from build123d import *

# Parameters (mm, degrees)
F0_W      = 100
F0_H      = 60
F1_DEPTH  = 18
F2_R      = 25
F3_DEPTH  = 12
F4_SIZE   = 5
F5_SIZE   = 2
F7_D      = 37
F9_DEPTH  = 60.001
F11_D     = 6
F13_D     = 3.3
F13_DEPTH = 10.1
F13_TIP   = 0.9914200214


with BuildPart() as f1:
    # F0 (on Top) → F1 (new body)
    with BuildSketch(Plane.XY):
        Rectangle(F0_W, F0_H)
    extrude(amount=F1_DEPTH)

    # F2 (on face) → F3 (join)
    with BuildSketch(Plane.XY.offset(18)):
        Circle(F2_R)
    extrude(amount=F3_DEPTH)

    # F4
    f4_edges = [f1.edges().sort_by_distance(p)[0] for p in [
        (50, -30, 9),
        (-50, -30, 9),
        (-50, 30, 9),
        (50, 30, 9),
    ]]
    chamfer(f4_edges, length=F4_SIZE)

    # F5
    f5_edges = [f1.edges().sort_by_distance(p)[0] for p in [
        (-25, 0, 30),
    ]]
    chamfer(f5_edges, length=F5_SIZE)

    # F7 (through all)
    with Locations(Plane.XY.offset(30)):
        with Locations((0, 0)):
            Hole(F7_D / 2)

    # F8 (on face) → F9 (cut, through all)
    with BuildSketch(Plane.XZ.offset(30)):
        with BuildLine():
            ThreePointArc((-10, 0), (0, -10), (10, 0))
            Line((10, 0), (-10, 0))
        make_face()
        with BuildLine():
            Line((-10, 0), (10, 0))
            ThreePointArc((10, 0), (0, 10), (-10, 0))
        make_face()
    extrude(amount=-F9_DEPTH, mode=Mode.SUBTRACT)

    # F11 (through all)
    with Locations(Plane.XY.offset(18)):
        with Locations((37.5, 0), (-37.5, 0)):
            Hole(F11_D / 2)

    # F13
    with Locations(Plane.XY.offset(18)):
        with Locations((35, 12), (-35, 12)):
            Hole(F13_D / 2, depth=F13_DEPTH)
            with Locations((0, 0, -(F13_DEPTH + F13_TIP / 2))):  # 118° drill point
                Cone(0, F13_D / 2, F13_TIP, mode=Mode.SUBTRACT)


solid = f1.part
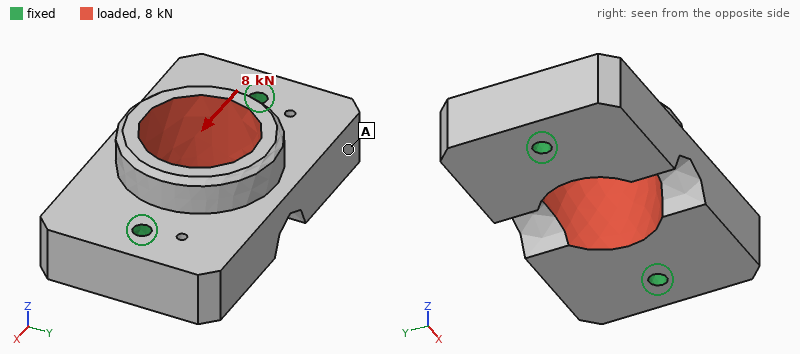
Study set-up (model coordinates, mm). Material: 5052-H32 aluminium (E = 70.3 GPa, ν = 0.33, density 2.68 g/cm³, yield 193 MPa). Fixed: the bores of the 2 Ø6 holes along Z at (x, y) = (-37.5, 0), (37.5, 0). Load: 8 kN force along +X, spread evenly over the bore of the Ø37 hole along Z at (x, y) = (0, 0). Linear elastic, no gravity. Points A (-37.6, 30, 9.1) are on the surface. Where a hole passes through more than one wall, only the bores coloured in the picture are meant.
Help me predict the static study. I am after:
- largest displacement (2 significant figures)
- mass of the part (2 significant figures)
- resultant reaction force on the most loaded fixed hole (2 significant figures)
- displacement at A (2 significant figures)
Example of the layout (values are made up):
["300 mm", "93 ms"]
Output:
["7.8 µm", "250 g", "4.1 kN", "3.7 µm"]
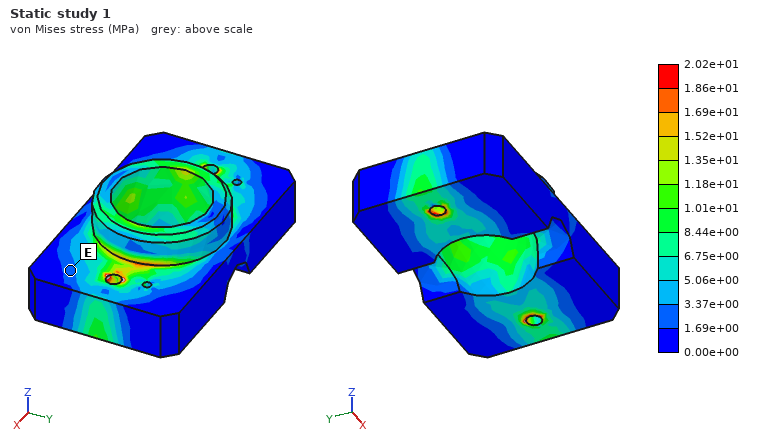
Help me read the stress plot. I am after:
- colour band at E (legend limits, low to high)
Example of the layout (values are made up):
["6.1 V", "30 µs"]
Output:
["1.69e+00 to 3.37e+00 MPa"]
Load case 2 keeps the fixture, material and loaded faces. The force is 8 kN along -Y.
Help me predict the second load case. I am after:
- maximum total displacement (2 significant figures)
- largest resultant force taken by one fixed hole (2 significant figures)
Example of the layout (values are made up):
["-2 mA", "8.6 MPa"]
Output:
["27 µm", "4.0 kN"]
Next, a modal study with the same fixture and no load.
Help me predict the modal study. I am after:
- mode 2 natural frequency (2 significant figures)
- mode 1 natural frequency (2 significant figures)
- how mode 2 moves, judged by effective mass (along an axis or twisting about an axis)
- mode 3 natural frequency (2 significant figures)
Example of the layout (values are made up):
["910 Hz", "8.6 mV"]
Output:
["9000 Hz", "7200 Hz", "along Z", "10 kHz"]
